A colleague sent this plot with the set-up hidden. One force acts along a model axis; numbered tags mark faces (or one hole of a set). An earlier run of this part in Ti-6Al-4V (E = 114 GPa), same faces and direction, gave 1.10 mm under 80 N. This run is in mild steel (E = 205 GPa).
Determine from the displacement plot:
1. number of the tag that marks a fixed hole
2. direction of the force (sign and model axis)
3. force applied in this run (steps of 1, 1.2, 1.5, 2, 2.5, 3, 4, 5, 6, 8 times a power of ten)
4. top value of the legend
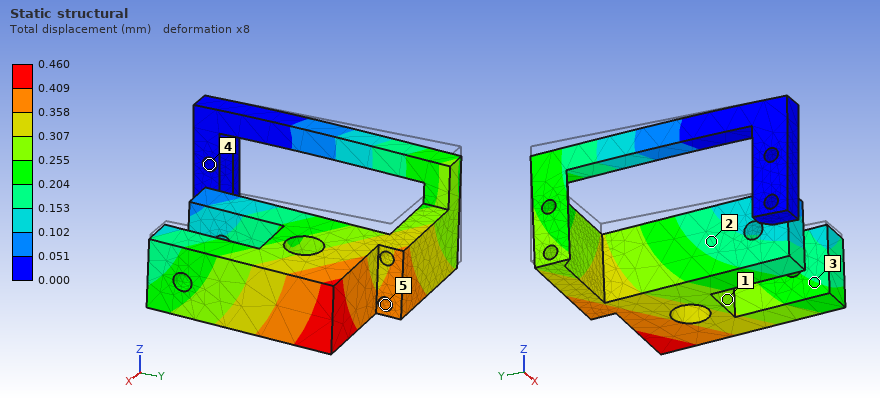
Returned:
4
-Z
60 N
0.460 mm
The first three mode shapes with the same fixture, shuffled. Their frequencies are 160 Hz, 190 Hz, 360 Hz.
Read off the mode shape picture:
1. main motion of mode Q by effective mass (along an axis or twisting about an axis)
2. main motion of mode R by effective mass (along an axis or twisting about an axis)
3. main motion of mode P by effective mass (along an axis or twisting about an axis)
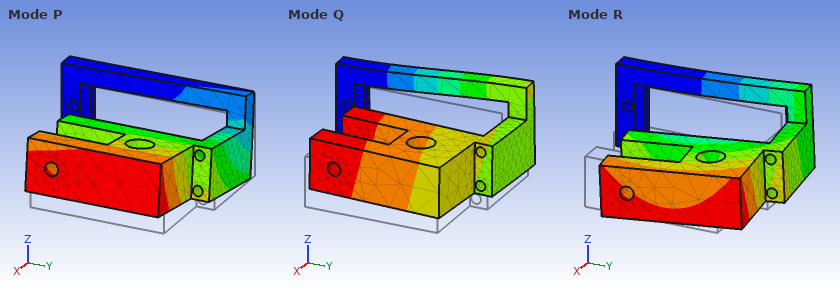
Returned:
along X
along Y
along Z
